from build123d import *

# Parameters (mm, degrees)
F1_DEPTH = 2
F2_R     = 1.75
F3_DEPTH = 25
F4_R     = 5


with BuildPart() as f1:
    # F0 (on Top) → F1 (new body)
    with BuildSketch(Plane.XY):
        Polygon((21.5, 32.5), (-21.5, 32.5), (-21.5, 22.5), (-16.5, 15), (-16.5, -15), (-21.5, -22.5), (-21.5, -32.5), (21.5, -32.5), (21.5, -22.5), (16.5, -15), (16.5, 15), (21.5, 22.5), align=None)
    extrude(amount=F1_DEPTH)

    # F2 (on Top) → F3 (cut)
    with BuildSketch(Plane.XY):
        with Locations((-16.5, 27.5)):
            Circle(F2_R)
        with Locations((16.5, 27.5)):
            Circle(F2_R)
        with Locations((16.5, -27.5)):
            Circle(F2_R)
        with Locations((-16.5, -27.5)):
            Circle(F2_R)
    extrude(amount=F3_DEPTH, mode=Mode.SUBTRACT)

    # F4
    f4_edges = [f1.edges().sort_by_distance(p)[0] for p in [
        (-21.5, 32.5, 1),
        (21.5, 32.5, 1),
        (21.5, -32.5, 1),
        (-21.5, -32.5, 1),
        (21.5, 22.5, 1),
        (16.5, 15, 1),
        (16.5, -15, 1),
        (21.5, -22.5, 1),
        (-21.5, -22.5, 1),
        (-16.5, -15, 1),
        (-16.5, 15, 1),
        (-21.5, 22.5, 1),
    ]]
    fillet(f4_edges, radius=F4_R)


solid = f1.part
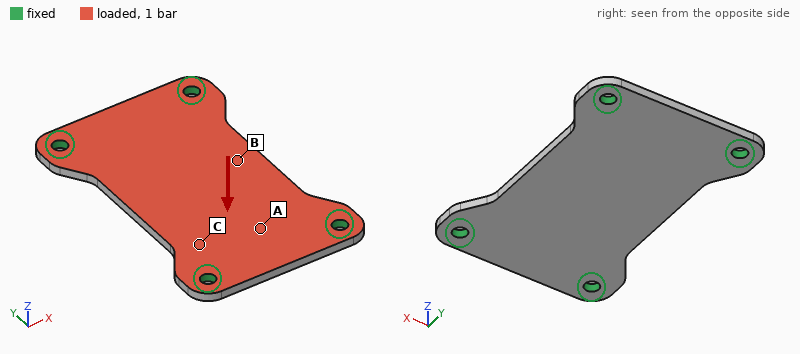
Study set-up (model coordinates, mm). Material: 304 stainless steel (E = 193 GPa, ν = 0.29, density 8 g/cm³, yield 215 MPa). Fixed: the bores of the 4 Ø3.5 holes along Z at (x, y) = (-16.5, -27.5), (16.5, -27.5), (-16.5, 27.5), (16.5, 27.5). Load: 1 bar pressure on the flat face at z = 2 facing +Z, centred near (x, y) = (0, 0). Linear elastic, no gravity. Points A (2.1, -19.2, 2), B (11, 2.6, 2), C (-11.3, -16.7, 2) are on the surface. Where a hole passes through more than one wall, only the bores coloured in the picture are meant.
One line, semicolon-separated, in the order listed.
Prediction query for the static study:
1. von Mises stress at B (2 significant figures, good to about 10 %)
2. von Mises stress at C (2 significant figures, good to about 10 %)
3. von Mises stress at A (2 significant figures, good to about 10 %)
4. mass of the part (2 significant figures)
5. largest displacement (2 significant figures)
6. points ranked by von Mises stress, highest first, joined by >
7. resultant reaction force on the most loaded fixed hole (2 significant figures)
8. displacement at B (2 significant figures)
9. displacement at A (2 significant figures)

18 MPa; 5.3 MPa; 10.0 MPa; 38 g; 21 µm; B > A > C; 59 N; 20 µm; 9.5 µm
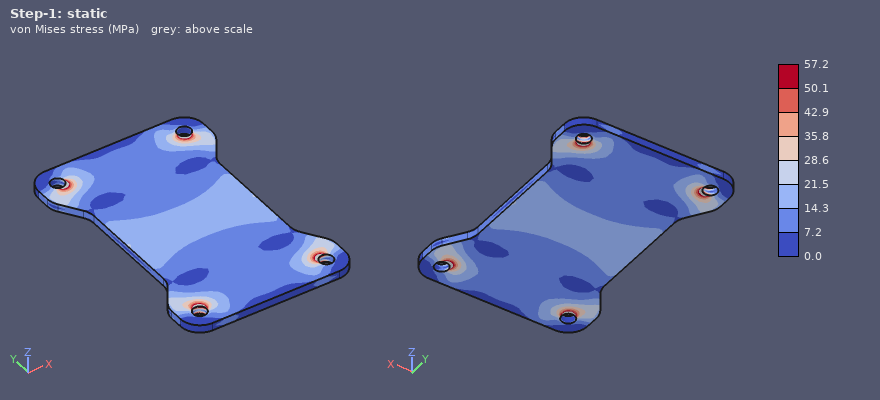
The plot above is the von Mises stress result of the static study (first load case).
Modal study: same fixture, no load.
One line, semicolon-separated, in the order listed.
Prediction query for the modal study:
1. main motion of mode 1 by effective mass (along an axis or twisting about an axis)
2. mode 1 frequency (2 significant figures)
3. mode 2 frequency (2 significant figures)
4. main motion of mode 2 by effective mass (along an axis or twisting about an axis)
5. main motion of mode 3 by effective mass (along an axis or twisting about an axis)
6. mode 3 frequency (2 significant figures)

along Z; 3100 Hz; 5600 Hz; twisting about Y; twisting about X; 7700 Hz
